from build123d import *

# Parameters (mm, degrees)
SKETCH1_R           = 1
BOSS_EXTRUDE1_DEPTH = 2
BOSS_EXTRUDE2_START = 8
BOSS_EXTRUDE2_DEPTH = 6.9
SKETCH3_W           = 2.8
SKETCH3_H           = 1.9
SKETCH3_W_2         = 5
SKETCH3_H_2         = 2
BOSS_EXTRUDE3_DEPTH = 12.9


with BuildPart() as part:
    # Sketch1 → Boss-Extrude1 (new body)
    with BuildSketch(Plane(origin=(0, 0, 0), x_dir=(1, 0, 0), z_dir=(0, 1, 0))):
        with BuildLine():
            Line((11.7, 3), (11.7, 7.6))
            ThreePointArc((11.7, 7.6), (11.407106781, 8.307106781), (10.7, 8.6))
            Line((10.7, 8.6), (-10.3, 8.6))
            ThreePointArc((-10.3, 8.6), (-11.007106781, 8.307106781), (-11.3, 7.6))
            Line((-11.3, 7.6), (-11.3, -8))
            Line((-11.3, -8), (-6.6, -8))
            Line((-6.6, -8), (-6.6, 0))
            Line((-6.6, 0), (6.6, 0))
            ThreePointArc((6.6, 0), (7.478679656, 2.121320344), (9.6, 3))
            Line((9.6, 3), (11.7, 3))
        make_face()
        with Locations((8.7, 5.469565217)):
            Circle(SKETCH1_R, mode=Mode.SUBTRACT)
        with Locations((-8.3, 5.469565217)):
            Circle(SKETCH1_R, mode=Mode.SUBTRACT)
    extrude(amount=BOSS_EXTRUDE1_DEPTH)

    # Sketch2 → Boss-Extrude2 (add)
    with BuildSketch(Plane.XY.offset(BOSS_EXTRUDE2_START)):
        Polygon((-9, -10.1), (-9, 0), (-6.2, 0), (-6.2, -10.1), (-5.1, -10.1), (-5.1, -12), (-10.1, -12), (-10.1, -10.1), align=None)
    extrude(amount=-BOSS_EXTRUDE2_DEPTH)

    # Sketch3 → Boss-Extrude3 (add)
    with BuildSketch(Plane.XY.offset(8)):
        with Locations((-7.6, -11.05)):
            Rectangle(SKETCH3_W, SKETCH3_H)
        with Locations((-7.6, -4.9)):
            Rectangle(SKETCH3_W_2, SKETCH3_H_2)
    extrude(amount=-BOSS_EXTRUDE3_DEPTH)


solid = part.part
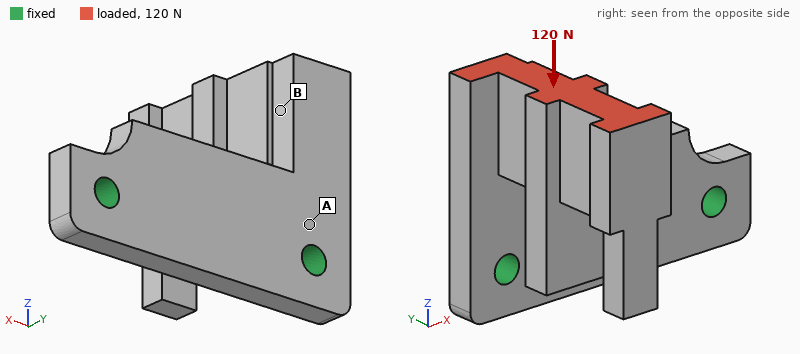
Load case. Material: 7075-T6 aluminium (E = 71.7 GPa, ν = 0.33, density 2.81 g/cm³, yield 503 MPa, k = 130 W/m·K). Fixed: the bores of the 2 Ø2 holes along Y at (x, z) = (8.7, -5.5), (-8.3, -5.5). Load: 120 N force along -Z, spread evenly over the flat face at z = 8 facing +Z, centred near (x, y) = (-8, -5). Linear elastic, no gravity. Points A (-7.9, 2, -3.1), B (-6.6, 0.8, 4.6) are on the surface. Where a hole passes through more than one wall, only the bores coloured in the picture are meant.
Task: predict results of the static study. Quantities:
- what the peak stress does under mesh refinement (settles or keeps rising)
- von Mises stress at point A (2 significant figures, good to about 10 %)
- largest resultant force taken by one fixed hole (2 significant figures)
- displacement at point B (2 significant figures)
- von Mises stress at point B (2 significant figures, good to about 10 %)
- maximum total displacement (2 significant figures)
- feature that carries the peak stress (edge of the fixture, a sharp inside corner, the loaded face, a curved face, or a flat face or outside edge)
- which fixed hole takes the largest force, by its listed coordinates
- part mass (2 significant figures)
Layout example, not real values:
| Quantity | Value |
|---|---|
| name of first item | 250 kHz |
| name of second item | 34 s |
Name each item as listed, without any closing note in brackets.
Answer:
| Quantity | Value |
|---|---|
| what the peak stress does under mesh refinement | keeps rising |
| von Mises stress at point A | 140 MPa |
| largest resultant force taken by one fixed hole | 120 N |
| displacement at point B | 0.11 mm |
| von Mises stress at point B | 42 MPa |
| maximum total displacement | 0.32 mm |
| feature that carries the peak stress | a sharp inside corner |
| which fixed hole takes the largest force, by its listed coordinates | (-8.3, -5.5) |
| part mass | 2.3 g |
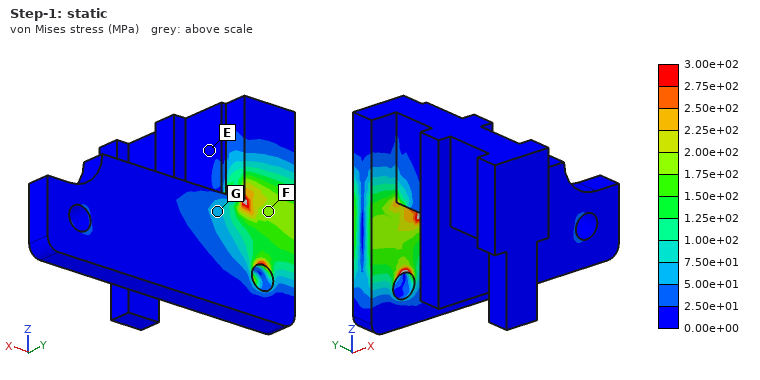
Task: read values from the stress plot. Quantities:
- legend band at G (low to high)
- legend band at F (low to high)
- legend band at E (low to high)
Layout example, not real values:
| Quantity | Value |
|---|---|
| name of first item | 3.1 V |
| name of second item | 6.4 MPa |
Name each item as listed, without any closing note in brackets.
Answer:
| Quantity | Value |
|---|---|
| legend band at G | 5.00e+01 to 7.50e+01 MPa |
| legend band at F | 1.75e+02 to 2.00e+02 MPa |
| legend band at E | 0.00e+00 to 2.50e+01 MPa |
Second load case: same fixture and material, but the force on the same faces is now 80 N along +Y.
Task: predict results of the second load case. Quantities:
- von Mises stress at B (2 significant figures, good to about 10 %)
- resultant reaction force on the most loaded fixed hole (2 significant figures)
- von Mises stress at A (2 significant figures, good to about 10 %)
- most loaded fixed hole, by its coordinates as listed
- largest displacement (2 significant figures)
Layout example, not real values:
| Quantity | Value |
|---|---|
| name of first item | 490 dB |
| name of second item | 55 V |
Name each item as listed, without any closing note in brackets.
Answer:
| Quantity | Value |
|---|---|
| von Mises stress at B | 33 MPa |
| resultant reaction force on the most loaded fixed hole | 86 N |
| von Mises stress at A | 190 MPa |
| most loaded fixed hole, by its coordinates as listed | (-8.3, -5.5) |
| largest displacement | 0.32 mm |
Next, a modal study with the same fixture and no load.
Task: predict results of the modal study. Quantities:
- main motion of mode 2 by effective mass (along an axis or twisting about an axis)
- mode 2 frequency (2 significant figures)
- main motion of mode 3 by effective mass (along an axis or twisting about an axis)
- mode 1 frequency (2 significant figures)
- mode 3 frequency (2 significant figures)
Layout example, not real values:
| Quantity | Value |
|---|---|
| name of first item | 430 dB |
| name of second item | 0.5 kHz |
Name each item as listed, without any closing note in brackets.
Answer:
| Quantity | Value |
|---|---|
| main motion of mode 2 by effective mass | along X |
| mode 2 frequency | 3600 Hz |
| main motion of mode 3 by effective mass | along Y |
| mode 1 frequency | 2900 Hz |
| mode 3 frequency | 12 kHz |
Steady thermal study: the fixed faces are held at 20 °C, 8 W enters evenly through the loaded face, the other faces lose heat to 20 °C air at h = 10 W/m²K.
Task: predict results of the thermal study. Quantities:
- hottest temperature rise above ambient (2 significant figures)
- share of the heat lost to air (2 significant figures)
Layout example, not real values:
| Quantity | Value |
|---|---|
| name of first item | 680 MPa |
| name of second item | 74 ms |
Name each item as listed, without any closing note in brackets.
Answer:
| Quantity | Value |
|---|---|
| hottest temperature rise above ambient | 63 K |
| share of the heat lost to air | 3.7 % |
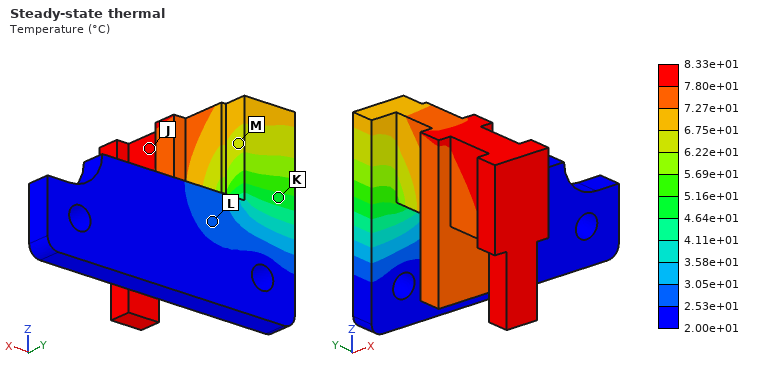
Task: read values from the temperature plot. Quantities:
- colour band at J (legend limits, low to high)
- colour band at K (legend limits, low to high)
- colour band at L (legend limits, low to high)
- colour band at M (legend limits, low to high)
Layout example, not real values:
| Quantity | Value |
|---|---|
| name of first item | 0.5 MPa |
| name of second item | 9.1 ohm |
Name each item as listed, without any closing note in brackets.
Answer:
| Quantity | Value |
|---|---|
| colour band at J | 7.80e+01 to 8.33e+01 °C |
| colour band at K | 4.64e+01 to 5.16e+01 °C |
| colour band at L | 2.53e+01 to 3.05e+01 °C |
| colour band at M | 6.22e+01 to 6.75e+01 °C |
